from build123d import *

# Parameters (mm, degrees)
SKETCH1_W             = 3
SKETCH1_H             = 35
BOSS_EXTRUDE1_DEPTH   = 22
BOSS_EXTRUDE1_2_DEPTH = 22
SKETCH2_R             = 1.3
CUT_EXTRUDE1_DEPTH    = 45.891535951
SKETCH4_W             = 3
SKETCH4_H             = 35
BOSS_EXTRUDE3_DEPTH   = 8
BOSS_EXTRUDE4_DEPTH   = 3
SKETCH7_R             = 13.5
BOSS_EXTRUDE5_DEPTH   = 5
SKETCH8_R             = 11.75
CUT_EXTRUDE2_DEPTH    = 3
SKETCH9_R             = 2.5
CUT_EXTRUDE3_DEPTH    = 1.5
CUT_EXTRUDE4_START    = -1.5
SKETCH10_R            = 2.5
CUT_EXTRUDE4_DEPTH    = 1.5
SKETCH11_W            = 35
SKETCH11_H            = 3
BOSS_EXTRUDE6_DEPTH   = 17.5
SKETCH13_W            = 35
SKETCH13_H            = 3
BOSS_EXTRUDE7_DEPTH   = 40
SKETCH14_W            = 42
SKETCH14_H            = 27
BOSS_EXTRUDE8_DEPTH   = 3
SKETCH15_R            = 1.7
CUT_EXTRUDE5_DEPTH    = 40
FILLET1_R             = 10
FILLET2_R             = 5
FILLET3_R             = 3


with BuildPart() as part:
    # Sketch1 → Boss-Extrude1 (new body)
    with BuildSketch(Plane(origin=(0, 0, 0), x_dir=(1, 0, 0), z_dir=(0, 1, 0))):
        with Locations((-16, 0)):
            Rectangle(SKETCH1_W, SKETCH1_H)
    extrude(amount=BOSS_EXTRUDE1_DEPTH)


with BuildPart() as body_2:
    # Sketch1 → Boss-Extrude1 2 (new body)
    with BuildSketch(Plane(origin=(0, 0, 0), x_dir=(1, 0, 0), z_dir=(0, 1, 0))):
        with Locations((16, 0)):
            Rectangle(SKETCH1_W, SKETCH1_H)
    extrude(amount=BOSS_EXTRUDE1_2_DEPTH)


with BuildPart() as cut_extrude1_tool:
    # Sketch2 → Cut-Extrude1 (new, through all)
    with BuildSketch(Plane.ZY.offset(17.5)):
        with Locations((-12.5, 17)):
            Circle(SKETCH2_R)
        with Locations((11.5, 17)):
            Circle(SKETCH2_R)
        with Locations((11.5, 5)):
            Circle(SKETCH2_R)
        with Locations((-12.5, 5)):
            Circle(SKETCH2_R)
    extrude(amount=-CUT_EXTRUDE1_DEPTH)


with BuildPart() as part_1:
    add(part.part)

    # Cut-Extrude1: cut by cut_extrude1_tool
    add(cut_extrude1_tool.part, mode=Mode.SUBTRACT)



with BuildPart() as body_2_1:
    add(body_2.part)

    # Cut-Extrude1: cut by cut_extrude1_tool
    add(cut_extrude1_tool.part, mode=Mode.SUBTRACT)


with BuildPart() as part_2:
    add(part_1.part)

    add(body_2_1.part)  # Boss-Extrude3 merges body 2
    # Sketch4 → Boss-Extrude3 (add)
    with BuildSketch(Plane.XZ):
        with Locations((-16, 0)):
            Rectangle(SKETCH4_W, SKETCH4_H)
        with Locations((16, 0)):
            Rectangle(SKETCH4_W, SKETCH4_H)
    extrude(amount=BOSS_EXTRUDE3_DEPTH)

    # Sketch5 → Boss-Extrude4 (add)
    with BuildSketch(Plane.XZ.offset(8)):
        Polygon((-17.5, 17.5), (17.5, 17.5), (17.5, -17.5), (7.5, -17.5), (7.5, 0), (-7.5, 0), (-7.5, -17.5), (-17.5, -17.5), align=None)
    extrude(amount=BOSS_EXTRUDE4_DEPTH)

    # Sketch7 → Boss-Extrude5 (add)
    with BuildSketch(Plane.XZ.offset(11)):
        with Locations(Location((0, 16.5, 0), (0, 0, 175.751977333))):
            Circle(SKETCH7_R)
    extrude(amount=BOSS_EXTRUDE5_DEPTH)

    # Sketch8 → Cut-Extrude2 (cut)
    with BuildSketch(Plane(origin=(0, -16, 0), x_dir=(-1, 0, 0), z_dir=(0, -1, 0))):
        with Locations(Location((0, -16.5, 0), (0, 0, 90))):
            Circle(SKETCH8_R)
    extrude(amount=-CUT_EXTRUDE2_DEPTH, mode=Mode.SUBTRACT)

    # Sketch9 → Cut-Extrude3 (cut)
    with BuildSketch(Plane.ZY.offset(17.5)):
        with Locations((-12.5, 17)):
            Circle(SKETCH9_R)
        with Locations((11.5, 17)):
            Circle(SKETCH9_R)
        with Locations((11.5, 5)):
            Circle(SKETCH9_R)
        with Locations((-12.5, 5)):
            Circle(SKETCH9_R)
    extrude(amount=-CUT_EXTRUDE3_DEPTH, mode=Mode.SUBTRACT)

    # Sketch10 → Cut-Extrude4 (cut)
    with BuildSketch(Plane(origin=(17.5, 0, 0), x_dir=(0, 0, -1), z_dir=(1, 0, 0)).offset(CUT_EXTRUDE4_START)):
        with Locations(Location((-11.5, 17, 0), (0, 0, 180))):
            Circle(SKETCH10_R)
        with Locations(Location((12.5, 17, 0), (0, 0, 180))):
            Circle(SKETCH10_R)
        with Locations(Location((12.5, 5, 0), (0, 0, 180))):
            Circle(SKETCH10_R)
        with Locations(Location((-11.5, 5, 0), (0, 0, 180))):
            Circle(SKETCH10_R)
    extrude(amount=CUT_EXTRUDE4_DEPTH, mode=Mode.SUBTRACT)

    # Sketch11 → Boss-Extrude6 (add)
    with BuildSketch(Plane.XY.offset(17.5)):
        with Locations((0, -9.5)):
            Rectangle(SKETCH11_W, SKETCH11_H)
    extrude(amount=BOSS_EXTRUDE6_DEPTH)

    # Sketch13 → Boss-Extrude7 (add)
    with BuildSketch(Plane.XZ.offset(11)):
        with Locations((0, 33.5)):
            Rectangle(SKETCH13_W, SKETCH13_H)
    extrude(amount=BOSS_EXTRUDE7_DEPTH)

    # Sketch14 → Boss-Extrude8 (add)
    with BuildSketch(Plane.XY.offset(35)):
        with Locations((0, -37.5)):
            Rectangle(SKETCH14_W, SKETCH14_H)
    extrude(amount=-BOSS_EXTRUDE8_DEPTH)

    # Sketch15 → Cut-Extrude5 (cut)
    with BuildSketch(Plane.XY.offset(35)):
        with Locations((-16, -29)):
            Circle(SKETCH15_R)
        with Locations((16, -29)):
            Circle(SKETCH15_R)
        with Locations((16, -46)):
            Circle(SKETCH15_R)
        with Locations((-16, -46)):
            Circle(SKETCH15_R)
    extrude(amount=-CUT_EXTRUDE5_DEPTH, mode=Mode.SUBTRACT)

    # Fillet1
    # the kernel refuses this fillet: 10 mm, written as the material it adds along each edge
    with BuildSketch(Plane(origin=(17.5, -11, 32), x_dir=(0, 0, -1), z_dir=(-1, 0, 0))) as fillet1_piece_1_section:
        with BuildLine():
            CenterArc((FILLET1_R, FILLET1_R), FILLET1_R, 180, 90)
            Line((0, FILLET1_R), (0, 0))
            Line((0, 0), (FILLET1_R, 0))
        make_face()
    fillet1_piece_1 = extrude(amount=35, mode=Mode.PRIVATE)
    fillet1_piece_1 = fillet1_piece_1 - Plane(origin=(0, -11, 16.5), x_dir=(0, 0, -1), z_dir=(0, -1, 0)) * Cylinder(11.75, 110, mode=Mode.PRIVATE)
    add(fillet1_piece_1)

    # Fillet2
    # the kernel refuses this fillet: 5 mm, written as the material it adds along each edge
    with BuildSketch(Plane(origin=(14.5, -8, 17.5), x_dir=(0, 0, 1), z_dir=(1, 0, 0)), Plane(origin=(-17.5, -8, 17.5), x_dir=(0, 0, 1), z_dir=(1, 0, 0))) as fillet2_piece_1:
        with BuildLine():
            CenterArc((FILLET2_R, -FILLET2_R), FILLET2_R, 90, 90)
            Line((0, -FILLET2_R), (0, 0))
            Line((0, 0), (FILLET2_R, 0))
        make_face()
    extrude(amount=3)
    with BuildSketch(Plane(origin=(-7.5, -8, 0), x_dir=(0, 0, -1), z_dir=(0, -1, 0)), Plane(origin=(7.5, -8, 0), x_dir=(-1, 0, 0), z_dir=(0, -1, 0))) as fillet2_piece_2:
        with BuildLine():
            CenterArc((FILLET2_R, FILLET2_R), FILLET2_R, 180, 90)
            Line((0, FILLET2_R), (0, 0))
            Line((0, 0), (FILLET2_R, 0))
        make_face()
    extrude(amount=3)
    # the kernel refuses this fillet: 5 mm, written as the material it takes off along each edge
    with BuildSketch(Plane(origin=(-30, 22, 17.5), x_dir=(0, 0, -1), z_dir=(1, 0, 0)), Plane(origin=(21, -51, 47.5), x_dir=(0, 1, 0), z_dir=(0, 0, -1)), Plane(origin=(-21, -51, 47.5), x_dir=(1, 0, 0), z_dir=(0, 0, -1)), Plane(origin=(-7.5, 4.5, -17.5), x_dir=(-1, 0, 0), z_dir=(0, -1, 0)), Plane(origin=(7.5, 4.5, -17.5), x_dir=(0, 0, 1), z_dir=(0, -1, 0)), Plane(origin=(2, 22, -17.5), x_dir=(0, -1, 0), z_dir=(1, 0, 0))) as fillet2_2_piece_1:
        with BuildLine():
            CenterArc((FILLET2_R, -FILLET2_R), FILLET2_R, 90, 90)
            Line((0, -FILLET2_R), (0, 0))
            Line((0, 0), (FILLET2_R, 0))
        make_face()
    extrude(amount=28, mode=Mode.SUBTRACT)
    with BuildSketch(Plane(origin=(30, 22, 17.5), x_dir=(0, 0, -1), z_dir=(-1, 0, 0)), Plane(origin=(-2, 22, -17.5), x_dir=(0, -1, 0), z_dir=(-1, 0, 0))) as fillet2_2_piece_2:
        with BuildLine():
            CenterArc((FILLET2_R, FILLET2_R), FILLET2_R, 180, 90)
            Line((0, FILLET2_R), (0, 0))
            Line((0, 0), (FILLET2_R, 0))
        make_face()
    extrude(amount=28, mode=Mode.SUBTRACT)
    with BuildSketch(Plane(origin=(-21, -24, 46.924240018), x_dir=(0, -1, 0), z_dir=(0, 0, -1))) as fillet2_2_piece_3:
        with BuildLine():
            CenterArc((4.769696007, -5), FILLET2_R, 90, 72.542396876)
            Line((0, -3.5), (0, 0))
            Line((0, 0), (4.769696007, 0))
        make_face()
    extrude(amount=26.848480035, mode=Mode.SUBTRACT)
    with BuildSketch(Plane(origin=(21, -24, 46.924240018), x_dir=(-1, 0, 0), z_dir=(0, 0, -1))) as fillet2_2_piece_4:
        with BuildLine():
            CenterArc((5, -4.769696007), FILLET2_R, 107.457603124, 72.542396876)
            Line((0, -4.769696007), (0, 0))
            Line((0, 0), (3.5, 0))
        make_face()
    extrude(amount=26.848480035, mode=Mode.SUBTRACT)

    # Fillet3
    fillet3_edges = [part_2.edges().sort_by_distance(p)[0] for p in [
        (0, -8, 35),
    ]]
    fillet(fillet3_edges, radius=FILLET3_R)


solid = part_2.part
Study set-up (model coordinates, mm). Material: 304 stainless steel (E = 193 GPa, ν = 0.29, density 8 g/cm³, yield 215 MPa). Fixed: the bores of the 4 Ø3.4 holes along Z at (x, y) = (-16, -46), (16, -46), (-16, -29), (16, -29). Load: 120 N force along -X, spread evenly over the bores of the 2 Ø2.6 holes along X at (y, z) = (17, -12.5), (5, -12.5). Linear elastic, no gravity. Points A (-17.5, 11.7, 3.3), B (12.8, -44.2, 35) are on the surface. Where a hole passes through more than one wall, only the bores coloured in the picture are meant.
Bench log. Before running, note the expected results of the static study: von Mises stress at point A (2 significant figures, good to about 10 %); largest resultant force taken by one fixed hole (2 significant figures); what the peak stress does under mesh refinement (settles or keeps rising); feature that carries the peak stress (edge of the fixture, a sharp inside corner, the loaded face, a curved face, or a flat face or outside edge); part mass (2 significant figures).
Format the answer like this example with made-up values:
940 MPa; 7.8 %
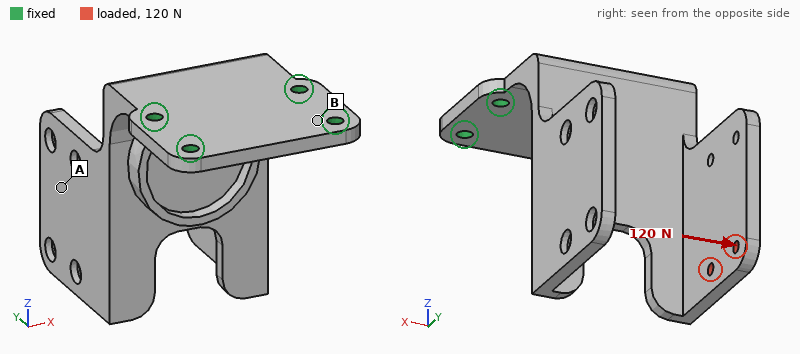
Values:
18 MPa; 250 N; keeps rising; edge of the fixture; 140 g
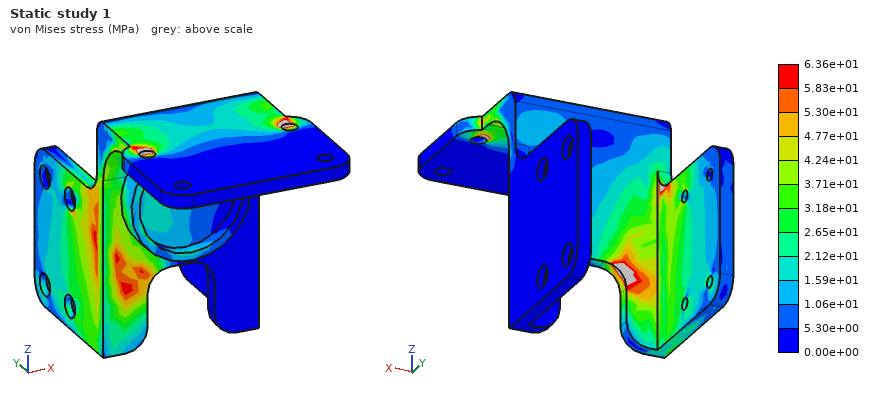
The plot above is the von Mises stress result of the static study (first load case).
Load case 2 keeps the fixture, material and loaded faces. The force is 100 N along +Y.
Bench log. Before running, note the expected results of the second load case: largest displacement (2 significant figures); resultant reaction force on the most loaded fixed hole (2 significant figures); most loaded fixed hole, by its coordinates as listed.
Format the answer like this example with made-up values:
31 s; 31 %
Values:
0.32 mm; 92 N; (-16, -29)
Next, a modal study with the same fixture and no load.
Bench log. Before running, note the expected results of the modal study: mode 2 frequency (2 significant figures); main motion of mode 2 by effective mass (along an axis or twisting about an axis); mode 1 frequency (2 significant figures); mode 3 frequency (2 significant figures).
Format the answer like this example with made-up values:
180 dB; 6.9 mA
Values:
1200 Hz; along X; 440 Hz; 1500 Hz
